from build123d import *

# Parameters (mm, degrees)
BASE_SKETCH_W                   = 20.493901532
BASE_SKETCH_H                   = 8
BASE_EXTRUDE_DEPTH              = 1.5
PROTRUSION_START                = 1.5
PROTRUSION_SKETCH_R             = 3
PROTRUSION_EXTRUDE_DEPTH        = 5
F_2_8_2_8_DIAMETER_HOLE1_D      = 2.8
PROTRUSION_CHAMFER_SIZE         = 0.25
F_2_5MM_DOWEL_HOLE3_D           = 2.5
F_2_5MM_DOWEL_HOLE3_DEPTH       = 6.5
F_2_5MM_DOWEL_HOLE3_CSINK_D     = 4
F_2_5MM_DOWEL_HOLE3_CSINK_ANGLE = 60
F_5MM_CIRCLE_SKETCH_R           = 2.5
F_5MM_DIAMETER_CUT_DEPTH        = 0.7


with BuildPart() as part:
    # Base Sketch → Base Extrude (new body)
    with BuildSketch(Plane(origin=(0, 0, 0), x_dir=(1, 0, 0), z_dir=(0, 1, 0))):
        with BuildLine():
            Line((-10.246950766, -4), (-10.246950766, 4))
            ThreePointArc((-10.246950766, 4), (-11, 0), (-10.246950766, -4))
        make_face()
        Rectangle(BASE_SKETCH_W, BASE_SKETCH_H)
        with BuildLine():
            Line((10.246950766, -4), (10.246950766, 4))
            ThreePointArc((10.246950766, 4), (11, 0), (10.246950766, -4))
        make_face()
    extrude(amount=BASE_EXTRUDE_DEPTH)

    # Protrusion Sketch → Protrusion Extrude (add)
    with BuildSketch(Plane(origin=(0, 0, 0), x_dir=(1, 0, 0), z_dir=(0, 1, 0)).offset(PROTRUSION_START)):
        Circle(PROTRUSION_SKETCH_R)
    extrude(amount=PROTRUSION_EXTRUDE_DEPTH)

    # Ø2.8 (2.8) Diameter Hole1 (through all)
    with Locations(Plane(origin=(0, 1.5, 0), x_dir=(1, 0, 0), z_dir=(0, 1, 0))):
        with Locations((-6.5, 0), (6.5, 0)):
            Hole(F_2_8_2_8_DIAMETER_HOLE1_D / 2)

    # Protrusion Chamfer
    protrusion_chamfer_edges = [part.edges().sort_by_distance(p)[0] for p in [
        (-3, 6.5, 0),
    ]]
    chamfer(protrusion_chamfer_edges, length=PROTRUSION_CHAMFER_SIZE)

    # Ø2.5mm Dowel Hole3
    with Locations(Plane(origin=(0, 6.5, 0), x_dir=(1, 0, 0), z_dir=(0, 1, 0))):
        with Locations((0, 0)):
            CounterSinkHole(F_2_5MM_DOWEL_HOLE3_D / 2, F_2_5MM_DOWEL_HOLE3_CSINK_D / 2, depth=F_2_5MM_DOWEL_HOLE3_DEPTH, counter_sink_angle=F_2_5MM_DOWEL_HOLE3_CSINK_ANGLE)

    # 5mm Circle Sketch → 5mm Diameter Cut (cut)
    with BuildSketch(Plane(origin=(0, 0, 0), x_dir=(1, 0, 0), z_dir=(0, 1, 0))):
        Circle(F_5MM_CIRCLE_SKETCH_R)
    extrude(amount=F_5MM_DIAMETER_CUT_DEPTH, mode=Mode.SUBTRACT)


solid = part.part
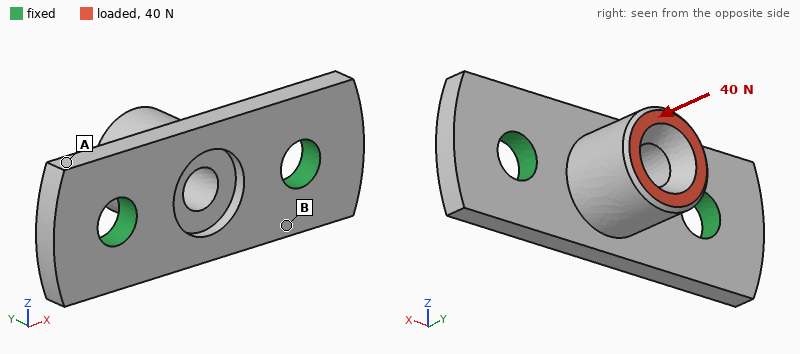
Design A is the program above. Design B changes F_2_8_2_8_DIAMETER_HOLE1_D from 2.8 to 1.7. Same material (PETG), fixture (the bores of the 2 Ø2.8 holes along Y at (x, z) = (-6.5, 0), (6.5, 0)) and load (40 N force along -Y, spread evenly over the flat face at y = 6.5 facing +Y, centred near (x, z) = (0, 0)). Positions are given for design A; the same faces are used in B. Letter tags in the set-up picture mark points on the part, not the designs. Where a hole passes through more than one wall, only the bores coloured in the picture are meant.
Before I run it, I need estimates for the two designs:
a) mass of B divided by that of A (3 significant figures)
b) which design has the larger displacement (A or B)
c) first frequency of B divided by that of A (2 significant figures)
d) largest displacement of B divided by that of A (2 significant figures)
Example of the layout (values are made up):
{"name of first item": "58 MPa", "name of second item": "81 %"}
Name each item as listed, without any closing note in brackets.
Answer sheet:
{"mass of B divided by that of A": "1.03", "which design has the larger displacement": "B", "first frequency of B divided by that of A": "0.85", "largest displacement of B divided by that of A": "1.5"}
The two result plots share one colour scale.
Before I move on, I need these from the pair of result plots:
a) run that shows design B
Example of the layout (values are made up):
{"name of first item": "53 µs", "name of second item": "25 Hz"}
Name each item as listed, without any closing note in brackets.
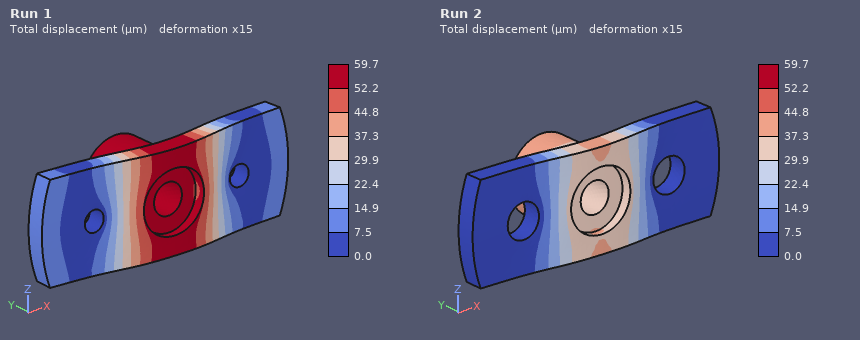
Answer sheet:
{"run that shows design B": "Run 1"}
